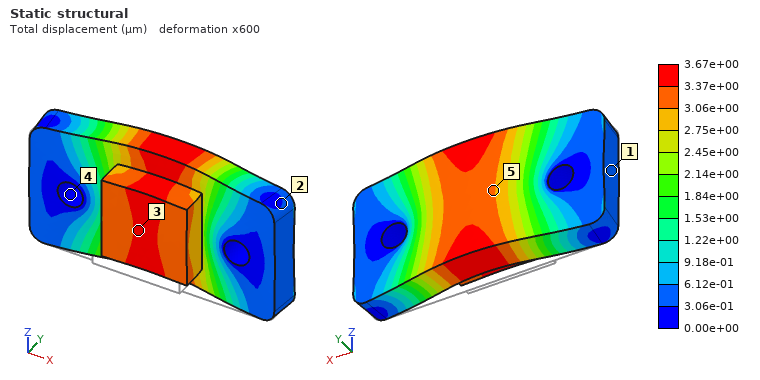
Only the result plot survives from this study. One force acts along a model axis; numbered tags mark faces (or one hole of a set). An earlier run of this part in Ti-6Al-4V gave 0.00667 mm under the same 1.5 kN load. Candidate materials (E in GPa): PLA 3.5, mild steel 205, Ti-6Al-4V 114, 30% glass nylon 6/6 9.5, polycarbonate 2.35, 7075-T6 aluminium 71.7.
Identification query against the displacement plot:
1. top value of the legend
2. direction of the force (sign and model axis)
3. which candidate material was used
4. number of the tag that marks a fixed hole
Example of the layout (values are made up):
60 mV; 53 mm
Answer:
3.67e+00 µm; +Y; mild steel; 4
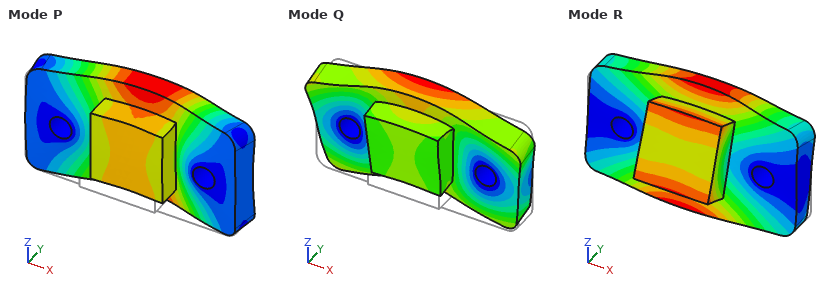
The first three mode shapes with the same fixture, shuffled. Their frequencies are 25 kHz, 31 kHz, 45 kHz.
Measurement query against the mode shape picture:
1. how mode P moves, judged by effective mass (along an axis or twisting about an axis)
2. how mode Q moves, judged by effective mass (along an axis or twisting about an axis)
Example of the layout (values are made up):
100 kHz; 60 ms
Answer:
along Y; along Z
